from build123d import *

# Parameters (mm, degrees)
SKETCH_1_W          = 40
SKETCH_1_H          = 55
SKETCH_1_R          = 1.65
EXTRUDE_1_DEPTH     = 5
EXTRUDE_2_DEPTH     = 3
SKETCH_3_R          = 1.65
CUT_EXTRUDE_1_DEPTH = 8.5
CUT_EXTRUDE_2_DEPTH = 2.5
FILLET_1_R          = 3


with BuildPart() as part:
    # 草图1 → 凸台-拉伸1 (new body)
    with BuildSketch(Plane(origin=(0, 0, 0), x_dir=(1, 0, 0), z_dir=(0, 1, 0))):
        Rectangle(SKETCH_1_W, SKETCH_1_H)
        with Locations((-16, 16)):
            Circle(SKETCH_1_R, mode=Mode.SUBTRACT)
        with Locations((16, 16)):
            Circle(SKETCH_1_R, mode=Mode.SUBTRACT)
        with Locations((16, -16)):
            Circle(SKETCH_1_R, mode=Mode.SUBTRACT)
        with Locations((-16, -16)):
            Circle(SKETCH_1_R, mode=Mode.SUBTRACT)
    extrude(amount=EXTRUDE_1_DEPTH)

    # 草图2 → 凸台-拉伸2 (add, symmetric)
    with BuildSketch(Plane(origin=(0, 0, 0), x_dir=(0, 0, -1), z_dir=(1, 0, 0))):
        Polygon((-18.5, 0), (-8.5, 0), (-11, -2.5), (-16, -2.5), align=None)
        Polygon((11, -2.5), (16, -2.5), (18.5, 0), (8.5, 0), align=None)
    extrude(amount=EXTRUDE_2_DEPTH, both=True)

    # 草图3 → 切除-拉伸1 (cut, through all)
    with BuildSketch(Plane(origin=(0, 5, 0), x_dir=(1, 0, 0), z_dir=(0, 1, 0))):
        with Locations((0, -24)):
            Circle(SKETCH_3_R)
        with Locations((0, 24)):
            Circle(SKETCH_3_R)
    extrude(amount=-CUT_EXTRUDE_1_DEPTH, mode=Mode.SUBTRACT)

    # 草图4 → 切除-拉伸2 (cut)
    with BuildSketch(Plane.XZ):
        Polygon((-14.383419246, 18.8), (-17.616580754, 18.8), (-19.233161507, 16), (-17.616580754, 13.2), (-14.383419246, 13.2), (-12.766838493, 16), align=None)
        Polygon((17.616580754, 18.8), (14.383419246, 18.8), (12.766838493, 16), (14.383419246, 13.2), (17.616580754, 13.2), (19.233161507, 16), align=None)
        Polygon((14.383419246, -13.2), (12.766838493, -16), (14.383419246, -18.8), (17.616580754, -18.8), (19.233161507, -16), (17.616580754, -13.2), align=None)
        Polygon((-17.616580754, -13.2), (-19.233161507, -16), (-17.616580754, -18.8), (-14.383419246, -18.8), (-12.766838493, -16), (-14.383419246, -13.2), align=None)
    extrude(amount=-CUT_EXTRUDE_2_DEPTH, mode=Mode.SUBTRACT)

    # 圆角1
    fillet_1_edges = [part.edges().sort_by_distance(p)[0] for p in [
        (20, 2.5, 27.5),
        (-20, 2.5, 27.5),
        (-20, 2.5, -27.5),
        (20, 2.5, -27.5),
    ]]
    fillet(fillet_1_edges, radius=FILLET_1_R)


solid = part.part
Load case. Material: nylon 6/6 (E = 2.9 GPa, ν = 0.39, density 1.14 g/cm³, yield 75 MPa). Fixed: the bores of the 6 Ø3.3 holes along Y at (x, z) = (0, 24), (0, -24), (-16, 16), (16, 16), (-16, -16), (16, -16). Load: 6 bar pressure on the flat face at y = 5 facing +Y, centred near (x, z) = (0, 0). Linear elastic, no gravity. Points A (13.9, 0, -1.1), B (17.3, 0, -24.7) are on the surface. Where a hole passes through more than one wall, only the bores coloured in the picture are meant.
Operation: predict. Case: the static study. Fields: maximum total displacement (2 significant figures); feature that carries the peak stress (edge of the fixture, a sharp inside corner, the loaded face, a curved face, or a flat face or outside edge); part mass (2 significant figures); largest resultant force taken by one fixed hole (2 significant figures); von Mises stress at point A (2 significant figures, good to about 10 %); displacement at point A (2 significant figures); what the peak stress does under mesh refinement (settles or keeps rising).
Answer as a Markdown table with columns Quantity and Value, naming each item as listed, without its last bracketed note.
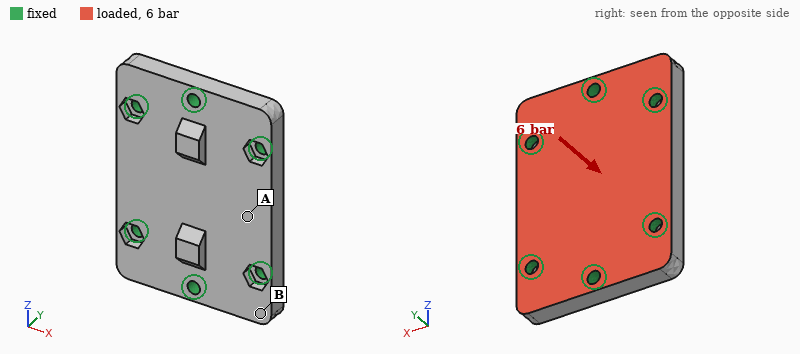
| Quantity | Value |
|---|---|
| maximum total displacement | 0.15 mm |
| feature that carries the peak stress | edge of the fixture |
| part mass | 12 g |
| largest resultant force taken by one fixed hole | 240 N |
| von Mises stress at point A | 9.5 MPa |
| displacement at point A | 0.12 mm |
| what the peak stress does under mesh refinement | keeps rising |
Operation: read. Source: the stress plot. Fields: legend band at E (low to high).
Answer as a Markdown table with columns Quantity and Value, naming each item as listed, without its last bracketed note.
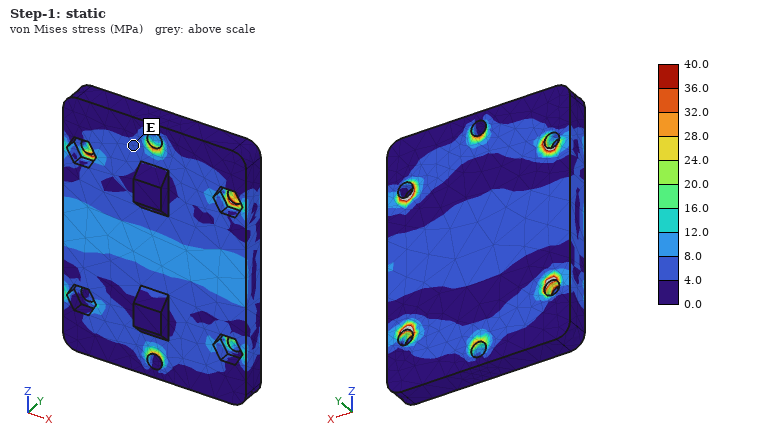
| Quantity | Value |
|---|---|
| legend band at E | 4.0 to 8.0 MPa |
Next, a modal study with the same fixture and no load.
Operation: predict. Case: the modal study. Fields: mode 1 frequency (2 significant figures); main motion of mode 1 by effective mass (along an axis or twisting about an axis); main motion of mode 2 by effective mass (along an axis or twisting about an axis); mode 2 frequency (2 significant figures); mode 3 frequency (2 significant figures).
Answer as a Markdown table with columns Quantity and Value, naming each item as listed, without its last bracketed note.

| Quantity | Value |
|---|---|
| mode 1 frequency | 4600 Hz |
| main motion of mode 1 by effective mass | along Y |
| main motion of mode 2 by effective mass | twisting about Z |
| mode 2 frequency | 6600 Hz |
| mode 3 frequency | 8900 Hz |
